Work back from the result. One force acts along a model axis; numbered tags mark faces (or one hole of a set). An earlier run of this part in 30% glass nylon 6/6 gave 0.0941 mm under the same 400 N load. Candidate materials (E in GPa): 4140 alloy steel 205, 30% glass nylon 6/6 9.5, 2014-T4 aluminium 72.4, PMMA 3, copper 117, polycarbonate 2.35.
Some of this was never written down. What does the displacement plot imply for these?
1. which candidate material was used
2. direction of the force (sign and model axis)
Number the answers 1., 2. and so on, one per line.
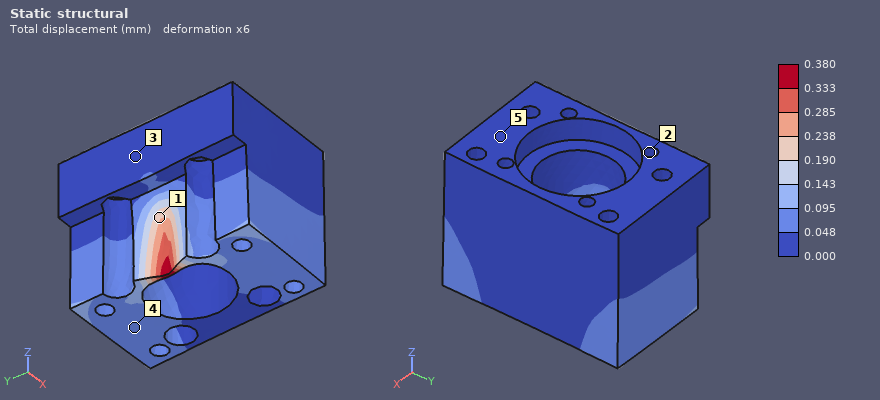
1. polycarbonate
2. +X
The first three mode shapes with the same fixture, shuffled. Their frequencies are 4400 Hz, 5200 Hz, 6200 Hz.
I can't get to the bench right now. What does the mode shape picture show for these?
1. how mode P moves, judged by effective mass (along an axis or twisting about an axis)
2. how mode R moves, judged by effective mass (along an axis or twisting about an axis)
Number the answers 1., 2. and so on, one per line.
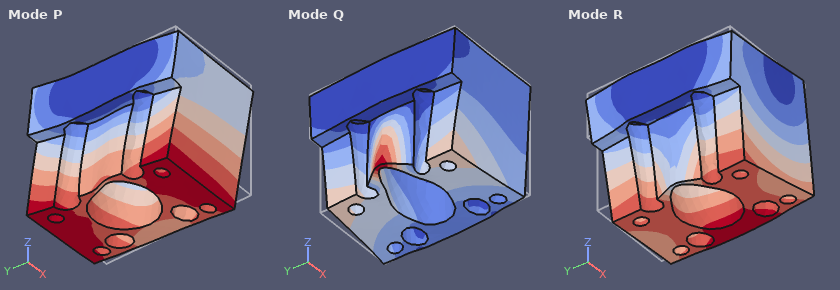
1. along Y
2. along X
